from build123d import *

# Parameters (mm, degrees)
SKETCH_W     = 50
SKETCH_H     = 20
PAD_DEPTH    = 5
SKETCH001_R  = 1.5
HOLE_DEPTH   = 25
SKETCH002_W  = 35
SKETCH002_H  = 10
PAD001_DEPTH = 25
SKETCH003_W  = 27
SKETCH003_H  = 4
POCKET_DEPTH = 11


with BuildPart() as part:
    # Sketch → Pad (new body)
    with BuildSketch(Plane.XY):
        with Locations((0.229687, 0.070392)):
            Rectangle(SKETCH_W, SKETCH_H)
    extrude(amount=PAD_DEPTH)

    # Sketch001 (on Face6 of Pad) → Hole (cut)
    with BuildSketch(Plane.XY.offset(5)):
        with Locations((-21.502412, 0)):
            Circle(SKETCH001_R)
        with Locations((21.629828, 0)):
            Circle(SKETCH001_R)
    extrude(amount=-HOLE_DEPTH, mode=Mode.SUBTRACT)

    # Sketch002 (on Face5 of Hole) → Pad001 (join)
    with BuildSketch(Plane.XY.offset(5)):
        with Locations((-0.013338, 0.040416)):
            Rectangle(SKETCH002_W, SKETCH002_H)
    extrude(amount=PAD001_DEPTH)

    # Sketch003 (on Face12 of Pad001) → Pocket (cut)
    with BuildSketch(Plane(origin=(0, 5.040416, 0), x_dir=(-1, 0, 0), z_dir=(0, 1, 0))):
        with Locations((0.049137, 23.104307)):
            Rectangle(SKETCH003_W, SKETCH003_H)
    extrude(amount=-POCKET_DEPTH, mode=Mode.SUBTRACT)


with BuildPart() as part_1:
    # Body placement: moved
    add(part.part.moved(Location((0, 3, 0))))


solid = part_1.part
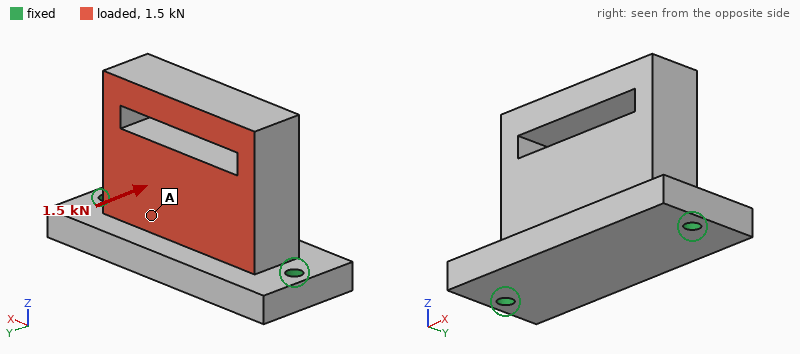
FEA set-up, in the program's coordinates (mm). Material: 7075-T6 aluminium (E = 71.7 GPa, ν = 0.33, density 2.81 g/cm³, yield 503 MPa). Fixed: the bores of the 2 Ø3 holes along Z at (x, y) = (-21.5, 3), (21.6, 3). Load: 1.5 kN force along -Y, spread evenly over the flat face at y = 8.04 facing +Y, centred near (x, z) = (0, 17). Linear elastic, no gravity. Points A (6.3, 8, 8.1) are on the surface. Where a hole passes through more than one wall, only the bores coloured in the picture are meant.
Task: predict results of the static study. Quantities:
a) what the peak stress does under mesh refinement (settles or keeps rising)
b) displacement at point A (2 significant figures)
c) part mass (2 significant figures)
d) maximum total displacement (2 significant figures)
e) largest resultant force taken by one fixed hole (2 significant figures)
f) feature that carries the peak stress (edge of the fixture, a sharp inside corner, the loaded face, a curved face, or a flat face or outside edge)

keeps rising
0.042 mm
35 g
0.16 mm
750 N
edge of the fixture
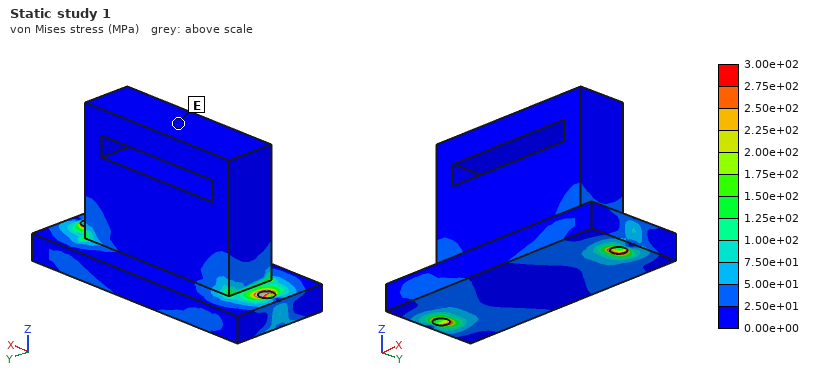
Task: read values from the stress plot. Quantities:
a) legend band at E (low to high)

0.00e+00 to 2.50e+01 MPa
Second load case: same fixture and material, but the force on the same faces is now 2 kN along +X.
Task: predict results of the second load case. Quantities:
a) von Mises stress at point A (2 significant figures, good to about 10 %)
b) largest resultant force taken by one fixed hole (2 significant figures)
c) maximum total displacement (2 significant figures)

20 MPa
1.3 kN
28 µm
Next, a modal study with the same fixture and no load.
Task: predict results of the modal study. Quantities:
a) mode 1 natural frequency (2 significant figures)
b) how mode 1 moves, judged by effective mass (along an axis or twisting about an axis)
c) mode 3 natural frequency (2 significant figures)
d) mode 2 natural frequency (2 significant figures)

4000 Hz
along Y
13 kHz
12 kHz
